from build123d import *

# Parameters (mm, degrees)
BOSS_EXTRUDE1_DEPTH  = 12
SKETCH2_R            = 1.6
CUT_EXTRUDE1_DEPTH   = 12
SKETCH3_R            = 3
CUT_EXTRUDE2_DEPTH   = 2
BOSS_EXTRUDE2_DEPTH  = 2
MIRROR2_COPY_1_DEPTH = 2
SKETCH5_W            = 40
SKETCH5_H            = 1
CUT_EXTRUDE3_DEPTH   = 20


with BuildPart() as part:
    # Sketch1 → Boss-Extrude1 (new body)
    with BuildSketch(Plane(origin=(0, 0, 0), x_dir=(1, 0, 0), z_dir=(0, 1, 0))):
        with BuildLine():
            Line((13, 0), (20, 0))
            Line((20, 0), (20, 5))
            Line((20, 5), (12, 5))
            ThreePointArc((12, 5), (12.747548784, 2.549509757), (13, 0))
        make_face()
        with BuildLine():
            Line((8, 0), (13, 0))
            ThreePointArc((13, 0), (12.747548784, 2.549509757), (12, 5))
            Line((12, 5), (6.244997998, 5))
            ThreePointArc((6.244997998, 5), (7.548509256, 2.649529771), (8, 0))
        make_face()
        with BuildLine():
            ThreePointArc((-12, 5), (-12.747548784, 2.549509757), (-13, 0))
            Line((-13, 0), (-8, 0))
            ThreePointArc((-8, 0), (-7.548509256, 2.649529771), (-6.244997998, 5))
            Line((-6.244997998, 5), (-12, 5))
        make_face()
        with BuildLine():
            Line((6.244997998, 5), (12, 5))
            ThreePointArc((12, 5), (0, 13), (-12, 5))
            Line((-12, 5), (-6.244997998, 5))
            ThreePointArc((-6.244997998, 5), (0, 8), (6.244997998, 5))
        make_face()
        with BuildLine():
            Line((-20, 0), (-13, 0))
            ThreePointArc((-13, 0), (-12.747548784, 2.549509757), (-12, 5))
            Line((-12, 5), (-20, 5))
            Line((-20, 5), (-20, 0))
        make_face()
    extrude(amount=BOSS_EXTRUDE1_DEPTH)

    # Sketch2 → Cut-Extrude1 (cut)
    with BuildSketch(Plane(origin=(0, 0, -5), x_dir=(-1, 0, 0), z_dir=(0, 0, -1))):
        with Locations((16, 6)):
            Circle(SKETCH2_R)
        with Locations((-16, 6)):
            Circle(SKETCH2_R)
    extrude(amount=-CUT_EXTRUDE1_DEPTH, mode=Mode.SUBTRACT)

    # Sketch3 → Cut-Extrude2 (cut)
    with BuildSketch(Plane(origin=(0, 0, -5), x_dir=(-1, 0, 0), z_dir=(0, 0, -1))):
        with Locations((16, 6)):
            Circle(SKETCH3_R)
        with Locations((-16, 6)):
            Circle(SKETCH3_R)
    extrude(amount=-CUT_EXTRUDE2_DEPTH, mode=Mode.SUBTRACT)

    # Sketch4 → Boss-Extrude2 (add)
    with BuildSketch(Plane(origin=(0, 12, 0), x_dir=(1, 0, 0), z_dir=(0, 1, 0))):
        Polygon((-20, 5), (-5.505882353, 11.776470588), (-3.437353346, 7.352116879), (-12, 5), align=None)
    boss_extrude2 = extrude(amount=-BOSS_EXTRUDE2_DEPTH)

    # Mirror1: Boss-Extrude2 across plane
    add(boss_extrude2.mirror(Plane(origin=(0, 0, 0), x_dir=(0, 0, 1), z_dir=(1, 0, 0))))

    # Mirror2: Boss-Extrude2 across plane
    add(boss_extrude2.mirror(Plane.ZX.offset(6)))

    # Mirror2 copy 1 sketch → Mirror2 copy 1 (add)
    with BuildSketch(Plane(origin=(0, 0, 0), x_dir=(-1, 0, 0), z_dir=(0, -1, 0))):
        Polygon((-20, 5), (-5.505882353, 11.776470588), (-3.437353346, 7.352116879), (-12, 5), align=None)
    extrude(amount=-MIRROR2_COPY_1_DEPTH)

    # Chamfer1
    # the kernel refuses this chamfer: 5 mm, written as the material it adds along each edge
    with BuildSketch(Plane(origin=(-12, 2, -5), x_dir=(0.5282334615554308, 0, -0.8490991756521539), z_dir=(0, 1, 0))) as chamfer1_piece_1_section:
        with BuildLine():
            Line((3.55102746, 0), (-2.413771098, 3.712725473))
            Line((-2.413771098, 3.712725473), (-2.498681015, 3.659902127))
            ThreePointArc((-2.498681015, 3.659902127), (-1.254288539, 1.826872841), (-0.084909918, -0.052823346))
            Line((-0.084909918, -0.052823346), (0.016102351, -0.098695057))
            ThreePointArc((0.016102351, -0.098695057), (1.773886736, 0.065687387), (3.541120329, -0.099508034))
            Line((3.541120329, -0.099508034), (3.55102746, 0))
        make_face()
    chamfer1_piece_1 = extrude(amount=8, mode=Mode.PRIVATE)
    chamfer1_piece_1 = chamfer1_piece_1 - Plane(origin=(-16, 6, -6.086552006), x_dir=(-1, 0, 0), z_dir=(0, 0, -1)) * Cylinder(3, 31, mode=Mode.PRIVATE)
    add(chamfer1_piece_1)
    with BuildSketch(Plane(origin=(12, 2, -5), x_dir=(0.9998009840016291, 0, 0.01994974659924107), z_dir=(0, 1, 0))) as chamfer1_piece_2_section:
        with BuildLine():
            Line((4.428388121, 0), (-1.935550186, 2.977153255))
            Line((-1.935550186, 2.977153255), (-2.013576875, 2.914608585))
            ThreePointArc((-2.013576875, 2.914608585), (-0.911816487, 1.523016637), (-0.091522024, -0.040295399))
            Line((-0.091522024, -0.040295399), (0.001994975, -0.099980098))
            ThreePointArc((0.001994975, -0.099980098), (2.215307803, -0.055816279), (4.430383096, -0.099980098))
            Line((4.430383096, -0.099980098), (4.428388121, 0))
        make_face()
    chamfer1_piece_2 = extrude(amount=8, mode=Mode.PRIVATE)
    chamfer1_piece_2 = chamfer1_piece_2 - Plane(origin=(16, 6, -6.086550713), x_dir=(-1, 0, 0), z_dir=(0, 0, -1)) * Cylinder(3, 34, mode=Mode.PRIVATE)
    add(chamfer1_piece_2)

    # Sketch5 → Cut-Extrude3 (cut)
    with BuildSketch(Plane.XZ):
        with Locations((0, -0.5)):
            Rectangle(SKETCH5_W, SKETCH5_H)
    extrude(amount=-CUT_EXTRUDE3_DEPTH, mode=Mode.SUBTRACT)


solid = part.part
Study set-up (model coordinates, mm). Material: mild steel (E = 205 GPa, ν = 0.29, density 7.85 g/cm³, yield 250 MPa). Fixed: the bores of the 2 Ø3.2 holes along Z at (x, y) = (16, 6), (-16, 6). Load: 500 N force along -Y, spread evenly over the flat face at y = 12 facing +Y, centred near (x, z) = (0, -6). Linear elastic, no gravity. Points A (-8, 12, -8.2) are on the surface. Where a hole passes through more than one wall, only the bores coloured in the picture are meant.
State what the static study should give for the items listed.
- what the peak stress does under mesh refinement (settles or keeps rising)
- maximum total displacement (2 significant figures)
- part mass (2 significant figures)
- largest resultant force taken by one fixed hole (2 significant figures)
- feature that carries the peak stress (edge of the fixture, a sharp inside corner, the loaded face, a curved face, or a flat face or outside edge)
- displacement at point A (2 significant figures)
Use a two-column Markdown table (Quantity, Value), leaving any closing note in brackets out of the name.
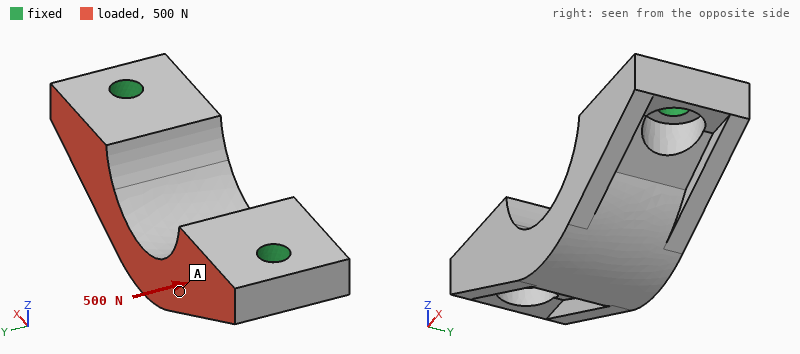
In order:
| Quantity | Value |
|---|---|
| what the peak stress does under mesh refinement | keeps rising |
| maximum total displacement | 8.7 µm |
| part mass | 21 g |
| largest resultant force taken by one fixed hole | 250 N |
| feature that carries the peak stress | edge of the fixture |
| displacement at point A | 5.8 µm |
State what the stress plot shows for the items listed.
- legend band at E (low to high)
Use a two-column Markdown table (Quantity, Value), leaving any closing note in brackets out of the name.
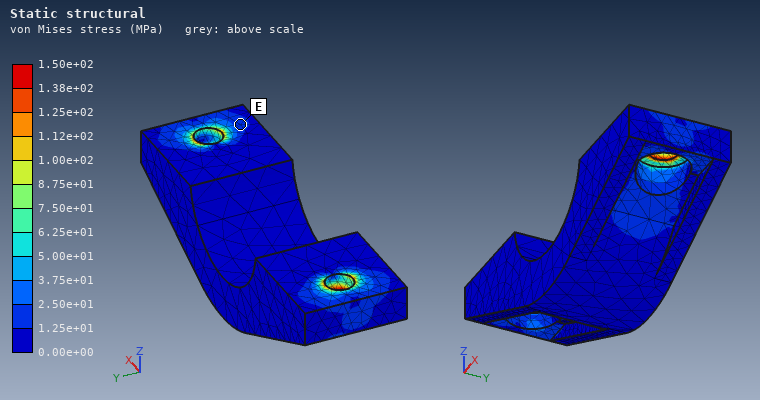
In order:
| Quantity | Value |
|---|---|
| legend band at E | 1.25e+01 to 2.50e+01 MPa |
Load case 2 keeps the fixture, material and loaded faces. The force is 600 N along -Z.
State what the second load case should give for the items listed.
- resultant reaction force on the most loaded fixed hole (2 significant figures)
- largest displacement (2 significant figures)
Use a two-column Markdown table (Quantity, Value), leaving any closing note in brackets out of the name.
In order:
| Quantity | Value |
|---|---|
| resultant reaction force on the most loaded fixed hole | 350 N |
| largest displacement | 12 µm |
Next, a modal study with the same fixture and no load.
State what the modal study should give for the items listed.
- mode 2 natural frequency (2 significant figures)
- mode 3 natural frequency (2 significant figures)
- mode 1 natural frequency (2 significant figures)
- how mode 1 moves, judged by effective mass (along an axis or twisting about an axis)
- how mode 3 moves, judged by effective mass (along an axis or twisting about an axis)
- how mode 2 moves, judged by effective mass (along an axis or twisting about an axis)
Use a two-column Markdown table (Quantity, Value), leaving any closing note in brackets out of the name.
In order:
| Quantity | Value |
|---|---|
| mode 2 natural frequency | 25 kHz |
| mode 3 natural frequency | 31 kHz |
| mode 1 natural frequency | 9900 Hz |
| how mode 1 moves, judged by effective mass | along Y |
| how mode 3 moves, judged by effective mass | along X |
| how mode 2 moves, judged by effective mass | along Z |
